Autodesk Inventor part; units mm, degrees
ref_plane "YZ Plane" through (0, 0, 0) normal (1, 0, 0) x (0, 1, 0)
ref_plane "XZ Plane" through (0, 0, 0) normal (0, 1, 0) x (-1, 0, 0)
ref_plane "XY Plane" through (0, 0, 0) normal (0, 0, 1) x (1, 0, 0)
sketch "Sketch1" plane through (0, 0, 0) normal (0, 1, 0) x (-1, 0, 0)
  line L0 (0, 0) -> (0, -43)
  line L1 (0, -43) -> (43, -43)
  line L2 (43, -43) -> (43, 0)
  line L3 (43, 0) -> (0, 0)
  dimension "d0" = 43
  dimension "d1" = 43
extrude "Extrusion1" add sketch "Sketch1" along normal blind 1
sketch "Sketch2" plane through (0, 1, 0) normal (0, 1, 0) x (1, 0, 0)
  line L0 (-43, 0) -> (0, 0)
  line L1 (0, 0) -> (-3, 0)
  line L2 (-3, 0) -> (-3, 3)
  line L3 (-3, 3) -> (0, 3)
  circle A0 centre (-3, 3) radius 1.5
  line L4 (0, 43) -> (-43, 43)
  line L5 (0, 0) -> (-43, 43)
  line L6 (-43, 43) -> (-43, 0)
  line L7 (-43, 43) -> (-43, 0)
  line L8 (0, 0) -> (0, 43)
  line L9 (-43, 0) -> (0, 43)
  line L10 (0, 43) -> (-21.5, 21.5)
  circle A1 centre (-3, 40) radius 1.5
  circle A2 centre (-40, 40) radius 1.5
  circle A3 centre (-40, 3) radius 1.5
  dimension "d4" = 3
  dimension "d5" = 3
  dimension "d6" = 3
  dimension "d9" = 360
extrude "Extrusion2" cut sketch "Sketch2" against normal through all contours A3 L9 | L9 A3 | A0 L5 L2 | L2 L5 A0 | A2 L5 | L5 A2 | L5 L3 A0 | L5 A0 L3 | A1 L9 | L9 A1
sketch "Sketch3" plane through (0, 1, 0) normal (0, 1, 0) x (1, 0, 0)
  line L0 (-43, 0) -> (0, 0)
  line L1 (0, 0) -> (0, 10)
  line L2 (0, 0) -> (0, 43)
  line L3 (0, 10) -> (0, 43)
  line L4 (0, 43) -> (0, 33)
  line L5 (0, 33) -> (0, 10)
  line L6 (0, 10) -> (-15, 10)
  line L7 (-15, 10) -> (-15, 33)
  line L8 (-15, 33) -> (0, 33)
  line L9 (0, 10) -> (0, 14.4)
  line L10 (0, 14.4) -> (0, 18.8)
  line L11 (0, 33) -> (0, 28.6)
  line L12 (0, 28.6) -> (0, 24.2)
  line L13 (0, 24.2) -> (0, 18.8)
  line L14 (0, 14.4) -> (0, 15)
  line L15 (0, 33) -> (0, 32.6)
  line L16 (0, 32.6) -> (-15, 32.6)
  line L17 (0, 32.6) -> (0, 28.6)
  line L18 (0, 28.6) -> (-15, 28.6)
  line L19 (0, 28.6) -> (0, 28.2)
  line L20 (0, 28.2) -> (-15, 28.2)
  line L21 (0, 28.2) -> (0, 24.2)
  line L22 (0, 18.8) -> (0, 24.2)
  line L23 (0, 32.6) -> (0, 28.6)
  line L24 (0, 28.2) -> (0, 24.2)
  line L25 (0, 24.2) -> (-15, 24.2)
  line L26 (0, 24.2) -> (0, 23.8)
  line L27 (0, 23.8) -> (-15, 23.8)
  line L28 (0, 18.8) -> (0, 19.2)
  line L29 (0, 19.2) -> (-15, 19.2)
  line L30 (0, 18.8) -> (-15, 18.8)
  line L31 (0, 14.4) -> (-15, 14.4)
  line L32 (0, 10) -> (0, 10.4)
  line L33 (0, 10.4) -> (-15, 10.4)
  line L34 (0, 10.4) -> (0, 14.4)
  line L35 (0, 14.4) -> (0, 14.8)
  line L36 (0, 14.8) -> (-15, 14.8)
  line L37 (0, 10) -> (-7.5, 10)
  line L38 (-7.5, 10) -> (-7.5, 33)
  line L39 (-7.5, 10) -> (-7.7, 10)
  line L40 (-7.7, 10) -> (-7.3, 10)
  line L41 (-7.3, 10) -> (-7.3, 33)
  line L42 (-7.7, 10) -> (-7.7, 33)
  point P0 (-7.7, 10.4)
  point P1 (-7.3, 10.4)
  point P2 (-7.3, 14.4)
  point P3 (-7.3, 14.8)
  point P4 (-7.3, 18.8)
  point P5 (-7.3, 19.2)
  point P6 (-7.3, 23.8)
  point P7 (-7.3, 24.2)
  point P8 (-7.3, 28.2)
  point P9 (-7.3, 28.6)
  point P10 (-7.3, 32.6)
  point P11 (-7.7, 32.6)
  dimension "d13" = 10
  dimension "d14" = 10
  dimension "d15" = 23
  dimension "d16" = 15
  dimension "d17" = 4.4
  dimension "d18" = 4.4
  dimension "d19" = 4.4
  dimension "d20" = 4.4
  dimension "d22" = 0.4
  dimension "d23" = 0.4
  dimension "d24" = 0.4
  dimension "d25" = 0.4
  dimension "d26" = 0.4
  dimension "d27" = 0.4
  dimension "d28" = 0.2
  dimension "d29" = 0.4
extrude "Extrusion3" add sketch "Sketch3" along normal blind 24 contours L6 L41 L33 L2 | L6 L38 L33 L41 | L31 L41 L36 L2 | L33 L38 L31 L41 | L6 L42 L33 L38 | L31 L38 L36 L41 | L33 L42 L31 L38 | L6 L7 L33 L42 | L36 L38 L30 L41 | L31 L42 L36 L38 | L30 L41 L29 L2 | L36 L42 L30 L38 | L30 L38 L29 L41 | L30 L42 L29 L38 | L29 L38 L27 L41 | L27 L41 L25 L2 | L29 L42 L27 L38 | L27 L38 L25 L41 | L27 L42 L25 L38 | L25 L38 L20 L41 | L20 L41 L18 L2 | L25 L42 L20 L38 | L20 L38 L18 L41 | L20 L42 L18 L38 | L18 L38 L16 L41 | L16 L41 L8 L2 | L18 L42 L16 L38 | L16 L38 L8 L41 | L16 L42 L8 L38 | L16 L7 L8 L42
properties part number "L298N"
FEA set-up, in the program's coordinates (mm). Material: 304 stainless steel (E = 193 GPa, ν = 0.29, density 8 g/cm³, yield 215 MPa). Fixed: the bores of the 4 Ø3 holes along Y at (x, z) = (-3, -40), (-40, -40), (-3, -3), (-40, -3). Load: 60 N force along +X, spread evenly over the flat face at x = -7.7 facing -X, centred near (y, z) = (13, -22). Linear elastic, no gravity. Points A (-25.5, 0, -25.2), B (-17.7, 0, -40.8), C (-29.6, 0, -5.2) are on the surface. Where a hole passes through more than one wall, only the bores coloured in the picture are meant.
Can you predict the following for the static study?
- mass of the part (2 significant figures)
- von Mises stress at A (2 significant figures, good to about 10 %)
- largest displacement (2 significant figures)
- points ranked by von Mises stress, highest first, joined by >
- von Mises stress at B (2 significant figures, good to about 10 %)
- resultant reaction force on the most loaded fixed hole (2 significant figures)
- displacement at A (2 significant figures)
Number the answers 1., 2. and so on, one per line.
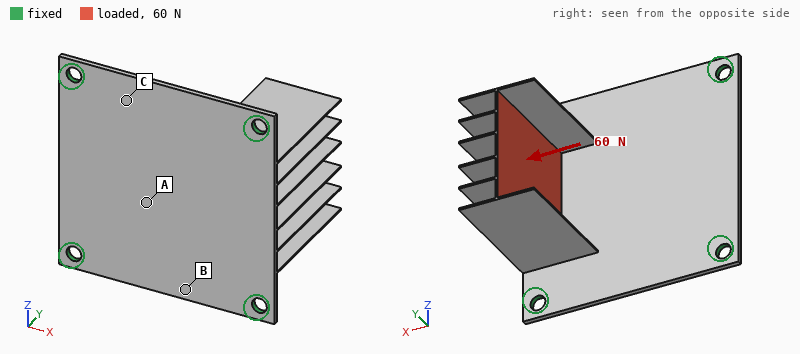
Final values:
1. 21 g
2. 14 MPa
3. 0.14 mm
4. B > A > C
5. 26 MPa
6. 22 N
7. 0.026 mm
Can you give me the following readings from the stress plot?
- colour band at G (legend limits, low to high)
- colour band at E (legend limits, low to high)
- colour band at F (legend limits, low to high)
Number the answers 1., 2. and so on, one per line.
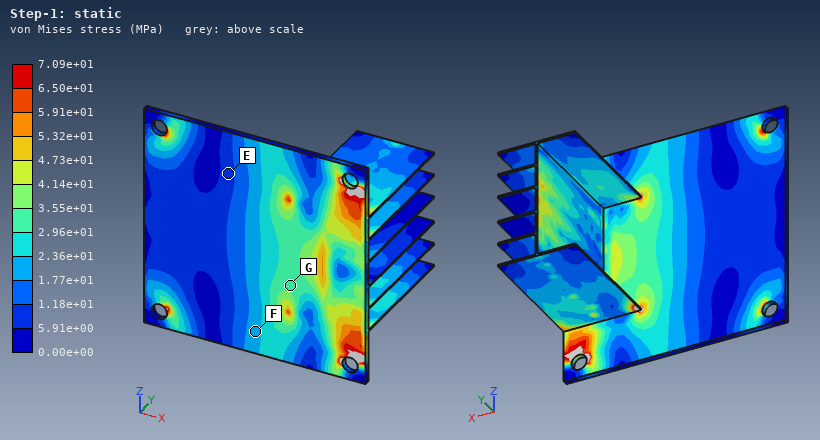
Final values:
1. 2.96e+01 to 3.55e+01 MPa
2. 5.91e+00 to 1.18e+01 MPa
3. 1.77e+01 to 2.36e+01 MPa
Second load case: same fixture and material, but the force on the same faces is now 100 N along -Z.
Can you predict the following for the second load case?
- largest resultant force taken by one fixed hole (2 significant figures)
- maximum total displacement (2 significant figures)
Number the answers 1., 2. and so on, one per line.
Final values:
1. 58 N
2. 27 µm
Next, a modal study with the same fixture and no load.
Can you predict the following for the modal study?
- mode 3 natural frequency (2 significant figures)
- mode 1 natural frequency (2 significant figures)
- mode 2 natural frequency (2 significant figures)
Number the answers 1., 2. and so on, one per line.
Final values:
1. 2900 Hz
2. 1700 Hz
3. 2900 Hz
